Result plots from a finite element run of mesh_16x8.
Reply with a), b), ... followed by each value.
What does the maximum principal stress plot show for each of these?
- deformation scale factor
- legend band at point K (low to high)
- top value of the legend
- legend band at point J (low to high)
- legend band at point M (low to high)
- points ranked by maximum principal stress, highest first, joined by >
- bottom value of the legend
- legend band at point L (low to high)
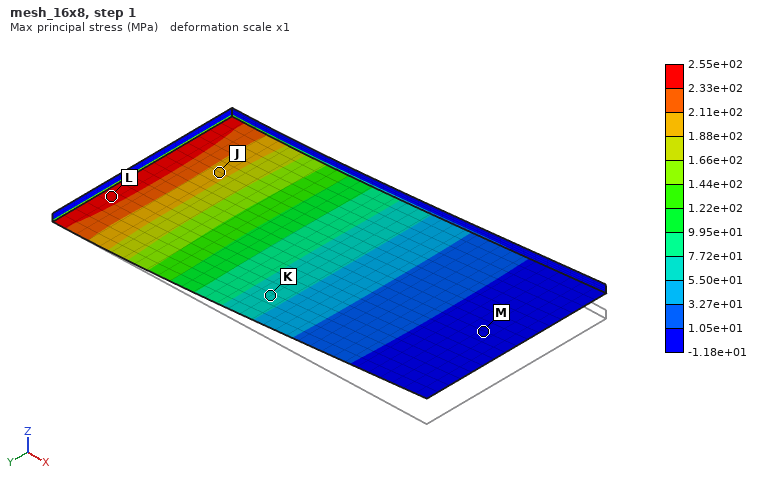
a) 1
b) 5.50e+01 to 7.72e+01 MPa
c) 2.55e+02 MPa
d) 1.88e+02 to 2.11e+02 MPa
e) -1.18e+01 to 1.05e+01 MPa
f) L > J > K > M
g) -1.18e+01 MPa
h) 2.33e+02 to 2.55e+02 MPa
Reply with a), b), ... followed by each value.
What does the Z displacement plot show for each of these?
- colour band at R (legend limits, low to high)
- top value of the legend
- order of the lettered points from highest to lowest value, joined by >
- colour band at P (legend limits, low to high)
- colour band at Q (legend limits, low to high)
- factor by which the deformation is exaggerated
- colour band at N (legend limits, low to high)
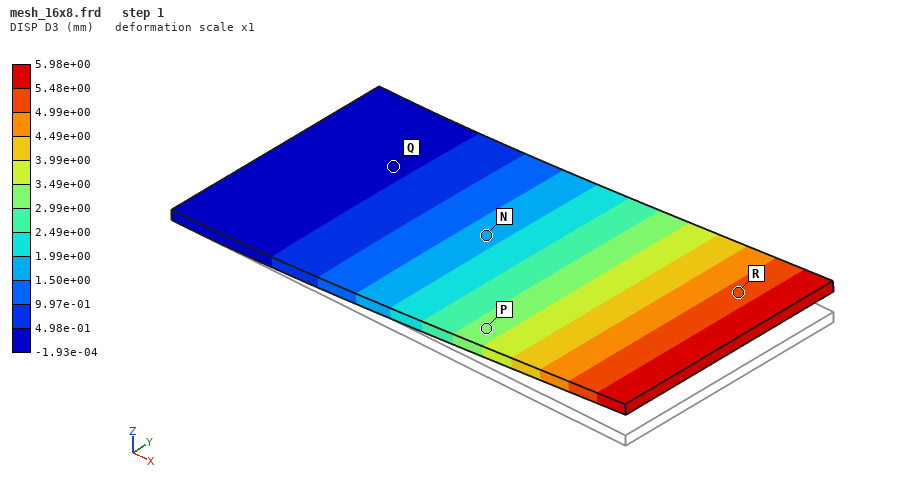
a) 4.99e+00 to 5.48e+00 mm
b) 5.98e+00 mm
c) R > P > N > Q
d) 2.99e+00 to 3.49e+00 mm
e) -1.93e-04 to 4.98e-01 mm
f) 1
g) 1.50e+00 to 1.99e+00 mm
